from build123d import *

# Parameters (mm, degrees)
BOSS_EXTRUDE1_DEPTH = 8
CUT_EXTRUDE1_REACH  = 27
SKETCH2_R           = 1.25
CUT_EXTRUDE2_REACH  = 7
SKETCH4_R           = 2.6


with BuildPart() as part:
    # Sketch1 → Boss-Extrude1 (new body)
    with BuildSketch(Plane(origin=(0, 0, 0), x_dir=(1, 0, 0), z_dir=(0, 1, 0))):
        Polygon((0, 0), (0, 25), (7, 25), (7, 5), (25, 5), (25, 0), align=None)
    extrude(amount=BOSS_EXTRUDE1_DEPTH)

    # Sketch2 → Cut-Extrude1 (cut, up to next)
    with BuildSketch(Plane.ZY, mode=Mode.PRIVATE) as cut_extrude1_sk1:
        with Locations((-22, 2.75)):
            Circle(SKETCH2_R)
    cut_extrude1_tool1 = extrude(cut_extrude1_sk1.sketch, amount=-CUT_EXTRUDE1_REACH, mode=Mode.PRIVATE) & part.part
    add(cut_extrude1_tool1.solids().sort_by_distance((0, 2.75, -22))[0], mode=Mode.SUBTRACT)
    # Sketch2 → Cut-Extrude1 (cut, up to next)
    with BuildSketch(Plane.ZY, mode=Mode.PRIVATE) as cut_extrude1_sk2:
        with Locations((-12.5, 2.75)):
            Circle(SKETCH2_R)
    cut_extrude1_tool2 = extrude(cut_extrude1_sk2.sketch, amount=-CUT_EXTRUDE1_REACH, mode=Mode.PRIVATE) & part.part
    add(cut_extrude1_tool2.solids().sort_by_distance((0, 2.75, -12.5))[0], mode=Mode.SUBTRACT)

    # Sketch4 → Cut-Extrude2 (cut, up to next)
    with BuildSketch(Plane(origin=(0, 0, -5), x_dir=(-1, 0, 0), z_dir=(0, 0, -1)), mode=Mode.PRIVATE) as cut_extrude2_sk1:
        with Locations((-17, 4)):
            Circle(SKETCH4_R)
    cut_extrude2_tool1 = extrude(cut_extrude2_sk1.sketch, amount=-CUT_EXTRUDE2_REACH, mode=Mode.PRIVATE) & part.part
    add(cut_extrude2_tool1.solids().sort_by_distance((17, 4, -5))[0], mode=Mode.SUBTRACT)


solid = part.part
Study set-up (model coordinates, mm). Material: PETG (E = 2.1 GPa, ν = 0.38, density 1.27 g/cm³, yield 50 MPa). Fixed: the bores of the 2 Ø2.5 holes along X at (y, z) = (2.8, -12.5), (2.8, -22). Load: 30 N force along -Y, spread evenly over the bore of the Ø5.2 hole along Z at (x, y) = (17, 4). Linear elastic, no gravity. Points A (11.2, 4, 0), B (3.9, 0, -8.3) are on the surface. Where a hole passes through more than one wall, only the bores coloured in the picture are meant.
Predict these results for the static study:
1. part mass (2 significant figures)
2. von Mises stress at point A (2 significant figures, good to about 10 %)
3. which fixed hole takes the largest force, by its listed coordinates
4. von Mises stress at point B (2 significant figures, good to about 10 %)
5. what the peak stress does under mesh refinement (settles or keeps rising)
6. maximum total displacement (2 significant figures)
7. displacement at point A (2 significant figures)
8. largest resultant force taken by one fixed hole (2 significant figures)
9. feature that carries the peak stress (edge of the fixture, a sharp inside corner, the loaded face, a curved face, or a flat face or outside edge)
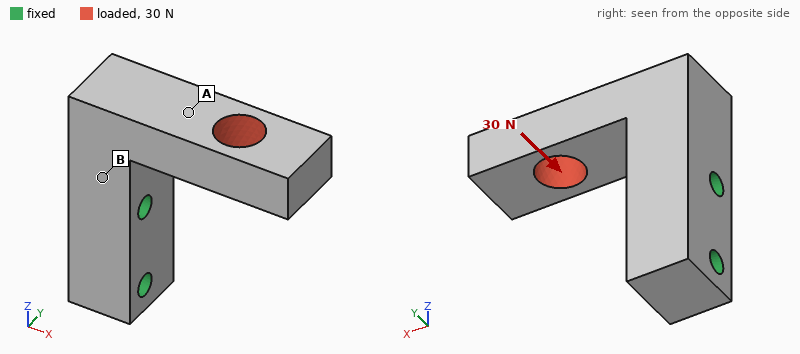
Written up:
2.5 g
2.4 MPa
(2.8, -12.5)
8.9 MPa
keeps rising
0.38 mm
0.14 mm
48 N
edge of the fixture
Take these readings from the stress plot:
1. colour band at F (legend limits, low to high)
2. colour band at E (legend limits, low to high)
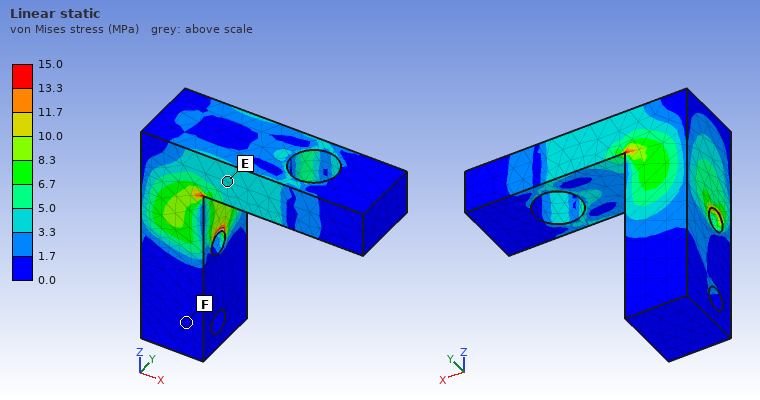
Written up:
0.0 to 1.7 MPa
3.3 to 5.0 MPa
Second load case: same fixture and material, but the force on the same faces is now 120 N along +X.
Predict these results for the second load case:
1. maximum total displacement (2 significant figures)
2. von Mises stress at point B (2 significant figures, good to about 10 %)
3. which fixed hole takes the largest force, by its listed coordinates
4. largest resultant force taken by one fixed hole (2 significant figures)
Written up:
0.36 mm
6.0 MPa
(2.8, -12.5)
140 N
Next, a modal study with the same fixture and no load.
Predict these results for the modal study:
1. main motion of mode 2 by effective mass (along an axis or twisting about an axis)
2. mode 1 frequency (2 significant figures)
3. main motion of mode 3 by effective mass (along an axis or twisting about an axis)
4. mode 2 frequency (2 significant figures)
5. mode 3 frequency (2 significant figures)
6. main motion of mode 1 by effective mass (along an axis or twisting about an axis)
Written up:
along Y
1900 Hz
along X
2000 Hz
5200 Hz
along Z
